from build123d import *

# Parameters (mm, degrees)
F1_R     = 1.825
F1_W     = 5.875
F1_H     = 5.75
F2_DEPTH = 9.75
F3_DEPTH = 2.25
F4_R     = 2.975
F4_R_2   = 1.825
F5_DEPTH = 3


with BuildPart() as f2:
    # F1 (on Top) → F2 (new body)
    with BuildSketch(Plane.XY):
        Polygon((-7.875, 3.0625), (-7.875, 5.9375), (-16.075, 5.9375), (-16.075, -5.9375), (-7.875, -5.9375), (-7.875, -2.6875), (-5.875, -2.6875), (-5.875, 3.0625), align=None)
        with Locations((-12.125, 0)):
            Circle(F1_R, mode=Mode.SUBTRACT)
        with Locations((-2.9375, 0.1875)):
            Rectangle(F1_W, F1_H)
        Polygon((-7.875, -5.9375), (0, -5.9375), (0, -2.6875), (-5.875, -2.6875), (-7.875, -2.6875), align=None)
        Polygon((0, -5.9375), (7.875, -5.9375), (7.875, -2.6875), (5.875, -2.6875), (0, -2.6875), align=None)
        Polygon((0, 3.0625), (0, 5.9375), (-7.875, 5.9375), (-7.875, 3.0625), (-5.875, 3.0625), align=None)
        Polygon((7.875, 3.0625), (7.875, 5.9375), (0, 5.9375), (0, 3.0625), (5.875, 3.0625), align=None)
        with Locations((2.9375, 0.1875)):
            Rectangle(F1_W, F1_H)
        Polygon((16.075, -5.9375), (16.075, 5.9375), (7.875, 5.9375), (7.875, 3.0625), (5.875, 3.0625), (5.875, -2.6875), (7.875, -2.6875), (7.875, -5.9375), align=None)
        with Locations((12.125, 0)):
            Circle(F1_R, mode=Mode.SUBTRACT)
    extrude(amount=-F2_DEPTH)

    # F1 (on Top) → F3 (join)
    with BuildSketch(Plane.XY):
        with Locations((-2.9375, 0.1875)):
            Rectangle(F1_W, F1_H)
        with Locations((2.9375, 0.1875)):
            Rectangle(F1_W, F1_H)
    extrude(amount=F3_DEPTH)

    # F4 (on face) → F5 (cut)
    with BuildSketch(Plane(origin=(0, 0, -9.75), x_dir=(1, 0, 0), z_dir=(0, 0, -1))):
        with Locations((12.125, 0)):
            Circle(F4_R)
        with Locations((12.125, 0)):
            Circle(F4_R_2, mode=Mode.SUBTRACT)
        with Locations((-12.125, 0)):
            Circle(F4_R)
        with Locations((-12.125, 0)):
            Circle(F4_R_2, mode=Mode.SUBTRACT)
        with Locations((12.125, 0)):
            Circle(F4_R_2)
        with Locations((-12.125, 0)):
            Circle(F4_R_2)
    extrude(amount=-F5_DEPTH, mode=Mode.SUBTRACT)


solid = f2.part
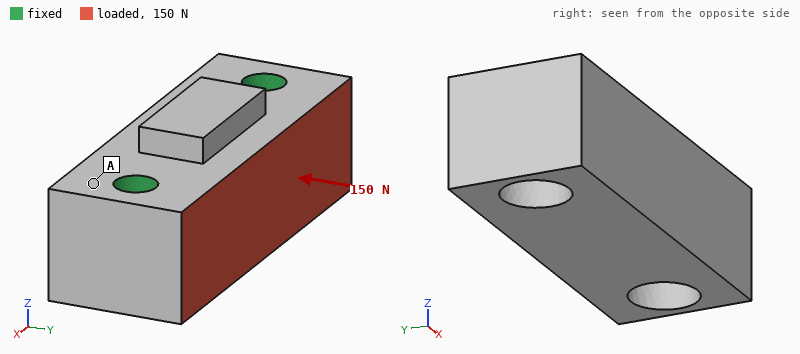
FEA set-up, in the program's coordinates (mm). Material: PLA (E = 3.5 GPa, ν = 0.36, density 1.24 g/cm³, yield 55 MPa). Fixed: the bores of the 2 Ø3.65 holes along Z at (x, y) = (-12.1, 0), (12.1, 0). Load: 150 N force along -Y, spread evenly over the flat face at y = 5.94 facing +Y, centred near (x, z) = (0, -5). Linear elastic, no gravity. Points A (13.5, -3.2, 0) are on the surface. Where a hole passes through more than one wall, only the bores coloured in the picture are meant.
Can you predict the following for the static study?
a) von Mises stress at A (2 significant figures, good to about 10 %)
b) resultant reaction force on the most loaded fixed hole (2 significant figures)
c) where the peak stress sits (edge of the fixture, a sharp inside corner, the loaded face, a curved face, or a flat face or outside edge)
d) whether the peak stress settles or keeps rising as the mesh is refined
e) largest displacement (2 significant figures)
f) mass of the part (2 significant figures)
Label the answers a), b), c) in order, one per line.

a) 0.44 MPa
b) 75 N
c) edge of the fixture
d) keeps rising
e) 7.2 µm
f) 4.4 g
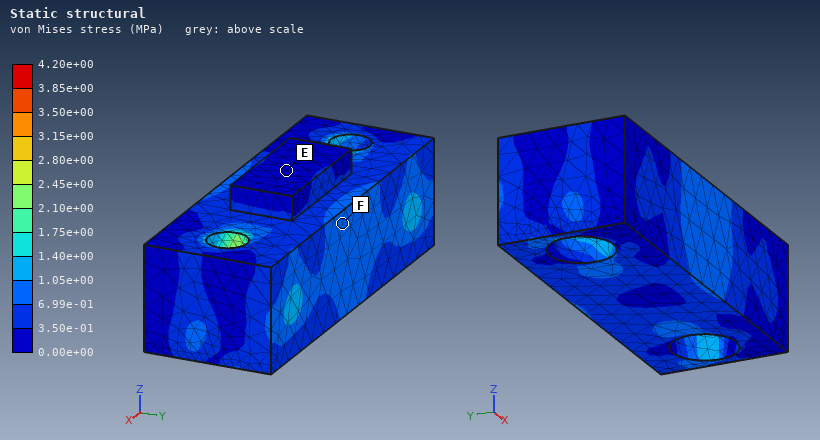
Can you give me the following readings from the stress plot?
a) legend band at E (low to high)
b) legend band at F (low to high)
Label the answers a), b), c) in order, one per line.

a) 0.00e+00 to 3.50e-01 MPa
b) 6.99e-01 to 1.05e+00 MPa
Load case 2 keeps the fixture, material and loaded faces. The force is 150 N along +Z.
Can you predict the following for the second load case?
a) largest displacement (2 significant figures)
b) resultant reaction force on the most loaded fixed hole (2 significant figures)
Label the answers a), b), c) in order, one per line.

a) 18 µm
b) 76 N
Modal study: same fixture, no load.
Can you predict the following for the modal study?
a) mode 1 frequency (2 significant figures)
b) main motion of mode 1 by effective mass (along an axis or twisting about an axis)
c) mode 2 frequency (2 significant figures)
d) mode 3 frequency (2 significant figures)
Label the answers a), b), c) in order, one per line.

a) 13 kHz
b) along Y
c) 14 kHz
d) 15 kHz
